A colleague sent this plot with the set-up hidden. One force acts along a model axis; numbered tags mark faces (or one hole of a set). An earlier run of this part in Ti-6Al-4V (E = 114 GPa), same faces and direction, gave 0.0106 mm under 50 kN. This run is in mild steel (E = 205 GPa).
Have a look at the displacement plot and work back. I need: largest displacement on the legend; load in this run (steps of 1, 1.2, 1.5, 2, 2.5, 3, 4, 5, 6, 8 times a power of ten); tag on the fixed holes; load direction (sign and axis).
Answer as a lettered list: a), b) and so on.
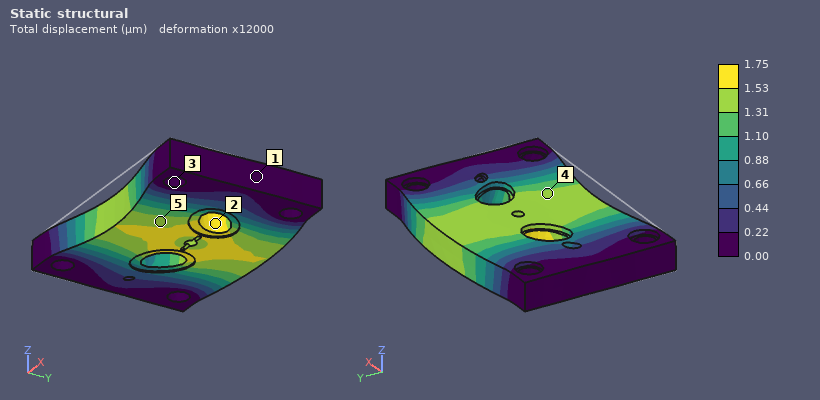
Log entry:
a) 1.75 µm
b) 15 kN
c) 3
d) +Y
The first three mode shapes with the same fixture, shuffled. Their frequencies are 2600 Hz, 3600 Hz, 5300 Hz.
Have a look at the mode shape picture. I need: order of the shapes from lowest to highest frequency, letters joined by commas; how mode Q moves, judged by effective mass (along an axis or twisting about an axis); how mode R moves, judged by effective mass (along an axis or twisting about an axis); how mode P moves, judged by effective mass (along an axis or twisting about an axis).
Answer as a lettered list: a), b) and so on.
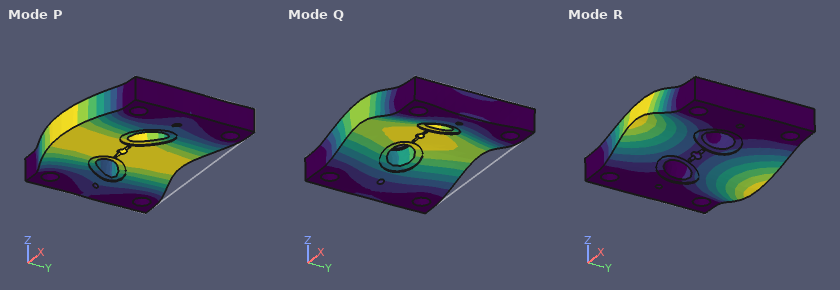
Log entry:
a) Q, R, P
b) along Z
c) twisting about X
d) along Y
